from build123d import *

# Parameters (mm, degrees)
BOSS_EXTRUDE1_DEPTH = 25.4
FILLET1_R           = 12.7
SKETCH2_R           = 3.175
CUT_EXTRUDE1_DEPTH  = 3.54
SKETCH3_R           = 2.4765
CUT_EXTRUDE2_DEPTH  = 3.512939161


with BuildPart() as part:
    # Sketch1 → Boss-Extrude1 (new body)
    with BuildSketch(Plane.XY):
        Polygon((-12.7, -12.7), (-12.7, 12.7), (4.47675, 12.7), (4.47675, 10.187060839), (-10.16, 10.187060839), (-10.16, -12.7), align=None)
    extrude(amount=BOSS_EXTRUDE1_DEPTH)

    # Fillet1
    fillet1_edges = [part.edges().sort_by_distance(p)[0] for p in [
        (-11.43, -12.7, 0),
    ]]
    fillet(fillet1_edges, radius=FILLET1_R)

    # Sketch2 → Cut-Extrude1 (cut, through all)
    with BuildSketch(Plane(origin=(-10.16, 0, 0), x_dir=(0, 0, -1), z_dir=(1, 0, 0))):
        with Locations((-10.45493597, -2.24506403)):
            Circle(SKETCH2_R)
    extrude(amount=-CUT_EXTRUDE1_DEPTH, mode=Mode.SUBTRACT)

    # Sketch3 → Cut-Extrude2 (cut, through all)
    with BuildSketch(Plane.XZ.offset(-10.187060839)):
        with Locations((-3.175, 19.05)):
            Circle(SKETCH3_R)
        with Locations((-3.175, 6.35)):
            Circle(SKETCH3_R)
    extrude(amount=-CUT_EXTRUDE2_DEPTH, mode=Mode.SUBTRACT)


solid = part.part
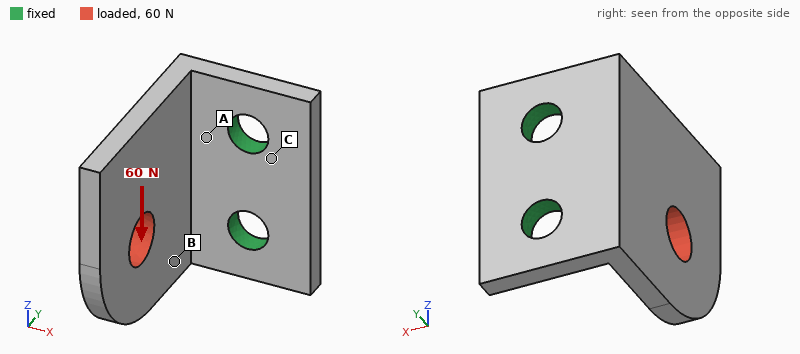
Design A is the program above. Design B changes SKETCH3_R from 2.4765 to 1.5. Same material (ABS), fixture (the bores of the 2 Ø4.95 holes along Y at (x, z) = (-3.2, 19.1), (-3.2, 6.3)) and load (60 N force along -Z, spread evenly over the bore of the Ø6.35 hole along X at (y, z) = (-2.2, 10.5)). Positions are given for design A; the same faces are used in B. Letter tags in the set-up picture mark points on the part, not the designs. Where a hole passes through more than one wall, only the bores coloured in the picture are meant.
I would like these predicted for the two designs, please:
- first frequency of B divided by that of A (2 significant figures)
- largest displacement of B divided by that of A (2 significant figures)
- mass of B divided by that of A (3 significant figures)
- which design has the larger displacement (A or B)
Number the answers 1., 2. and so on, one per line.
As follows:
1. 0.94
2. 1.4
3. 1.03
4. B
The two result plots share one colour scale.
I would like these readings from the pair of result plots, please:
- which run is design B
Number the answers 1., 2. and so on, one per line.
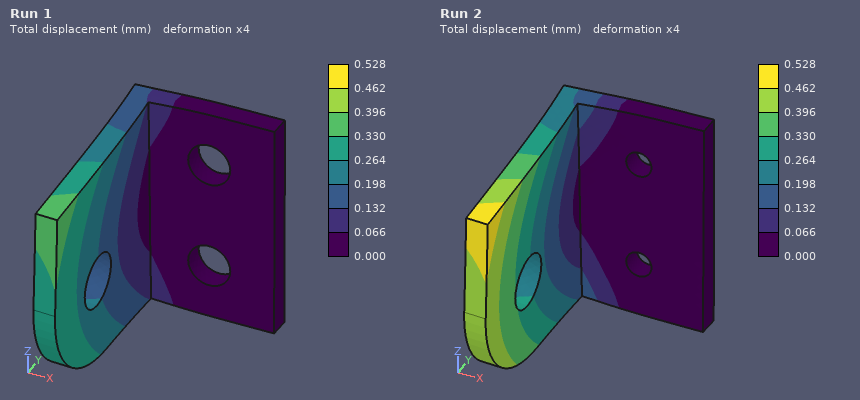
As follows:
1. Run 2
